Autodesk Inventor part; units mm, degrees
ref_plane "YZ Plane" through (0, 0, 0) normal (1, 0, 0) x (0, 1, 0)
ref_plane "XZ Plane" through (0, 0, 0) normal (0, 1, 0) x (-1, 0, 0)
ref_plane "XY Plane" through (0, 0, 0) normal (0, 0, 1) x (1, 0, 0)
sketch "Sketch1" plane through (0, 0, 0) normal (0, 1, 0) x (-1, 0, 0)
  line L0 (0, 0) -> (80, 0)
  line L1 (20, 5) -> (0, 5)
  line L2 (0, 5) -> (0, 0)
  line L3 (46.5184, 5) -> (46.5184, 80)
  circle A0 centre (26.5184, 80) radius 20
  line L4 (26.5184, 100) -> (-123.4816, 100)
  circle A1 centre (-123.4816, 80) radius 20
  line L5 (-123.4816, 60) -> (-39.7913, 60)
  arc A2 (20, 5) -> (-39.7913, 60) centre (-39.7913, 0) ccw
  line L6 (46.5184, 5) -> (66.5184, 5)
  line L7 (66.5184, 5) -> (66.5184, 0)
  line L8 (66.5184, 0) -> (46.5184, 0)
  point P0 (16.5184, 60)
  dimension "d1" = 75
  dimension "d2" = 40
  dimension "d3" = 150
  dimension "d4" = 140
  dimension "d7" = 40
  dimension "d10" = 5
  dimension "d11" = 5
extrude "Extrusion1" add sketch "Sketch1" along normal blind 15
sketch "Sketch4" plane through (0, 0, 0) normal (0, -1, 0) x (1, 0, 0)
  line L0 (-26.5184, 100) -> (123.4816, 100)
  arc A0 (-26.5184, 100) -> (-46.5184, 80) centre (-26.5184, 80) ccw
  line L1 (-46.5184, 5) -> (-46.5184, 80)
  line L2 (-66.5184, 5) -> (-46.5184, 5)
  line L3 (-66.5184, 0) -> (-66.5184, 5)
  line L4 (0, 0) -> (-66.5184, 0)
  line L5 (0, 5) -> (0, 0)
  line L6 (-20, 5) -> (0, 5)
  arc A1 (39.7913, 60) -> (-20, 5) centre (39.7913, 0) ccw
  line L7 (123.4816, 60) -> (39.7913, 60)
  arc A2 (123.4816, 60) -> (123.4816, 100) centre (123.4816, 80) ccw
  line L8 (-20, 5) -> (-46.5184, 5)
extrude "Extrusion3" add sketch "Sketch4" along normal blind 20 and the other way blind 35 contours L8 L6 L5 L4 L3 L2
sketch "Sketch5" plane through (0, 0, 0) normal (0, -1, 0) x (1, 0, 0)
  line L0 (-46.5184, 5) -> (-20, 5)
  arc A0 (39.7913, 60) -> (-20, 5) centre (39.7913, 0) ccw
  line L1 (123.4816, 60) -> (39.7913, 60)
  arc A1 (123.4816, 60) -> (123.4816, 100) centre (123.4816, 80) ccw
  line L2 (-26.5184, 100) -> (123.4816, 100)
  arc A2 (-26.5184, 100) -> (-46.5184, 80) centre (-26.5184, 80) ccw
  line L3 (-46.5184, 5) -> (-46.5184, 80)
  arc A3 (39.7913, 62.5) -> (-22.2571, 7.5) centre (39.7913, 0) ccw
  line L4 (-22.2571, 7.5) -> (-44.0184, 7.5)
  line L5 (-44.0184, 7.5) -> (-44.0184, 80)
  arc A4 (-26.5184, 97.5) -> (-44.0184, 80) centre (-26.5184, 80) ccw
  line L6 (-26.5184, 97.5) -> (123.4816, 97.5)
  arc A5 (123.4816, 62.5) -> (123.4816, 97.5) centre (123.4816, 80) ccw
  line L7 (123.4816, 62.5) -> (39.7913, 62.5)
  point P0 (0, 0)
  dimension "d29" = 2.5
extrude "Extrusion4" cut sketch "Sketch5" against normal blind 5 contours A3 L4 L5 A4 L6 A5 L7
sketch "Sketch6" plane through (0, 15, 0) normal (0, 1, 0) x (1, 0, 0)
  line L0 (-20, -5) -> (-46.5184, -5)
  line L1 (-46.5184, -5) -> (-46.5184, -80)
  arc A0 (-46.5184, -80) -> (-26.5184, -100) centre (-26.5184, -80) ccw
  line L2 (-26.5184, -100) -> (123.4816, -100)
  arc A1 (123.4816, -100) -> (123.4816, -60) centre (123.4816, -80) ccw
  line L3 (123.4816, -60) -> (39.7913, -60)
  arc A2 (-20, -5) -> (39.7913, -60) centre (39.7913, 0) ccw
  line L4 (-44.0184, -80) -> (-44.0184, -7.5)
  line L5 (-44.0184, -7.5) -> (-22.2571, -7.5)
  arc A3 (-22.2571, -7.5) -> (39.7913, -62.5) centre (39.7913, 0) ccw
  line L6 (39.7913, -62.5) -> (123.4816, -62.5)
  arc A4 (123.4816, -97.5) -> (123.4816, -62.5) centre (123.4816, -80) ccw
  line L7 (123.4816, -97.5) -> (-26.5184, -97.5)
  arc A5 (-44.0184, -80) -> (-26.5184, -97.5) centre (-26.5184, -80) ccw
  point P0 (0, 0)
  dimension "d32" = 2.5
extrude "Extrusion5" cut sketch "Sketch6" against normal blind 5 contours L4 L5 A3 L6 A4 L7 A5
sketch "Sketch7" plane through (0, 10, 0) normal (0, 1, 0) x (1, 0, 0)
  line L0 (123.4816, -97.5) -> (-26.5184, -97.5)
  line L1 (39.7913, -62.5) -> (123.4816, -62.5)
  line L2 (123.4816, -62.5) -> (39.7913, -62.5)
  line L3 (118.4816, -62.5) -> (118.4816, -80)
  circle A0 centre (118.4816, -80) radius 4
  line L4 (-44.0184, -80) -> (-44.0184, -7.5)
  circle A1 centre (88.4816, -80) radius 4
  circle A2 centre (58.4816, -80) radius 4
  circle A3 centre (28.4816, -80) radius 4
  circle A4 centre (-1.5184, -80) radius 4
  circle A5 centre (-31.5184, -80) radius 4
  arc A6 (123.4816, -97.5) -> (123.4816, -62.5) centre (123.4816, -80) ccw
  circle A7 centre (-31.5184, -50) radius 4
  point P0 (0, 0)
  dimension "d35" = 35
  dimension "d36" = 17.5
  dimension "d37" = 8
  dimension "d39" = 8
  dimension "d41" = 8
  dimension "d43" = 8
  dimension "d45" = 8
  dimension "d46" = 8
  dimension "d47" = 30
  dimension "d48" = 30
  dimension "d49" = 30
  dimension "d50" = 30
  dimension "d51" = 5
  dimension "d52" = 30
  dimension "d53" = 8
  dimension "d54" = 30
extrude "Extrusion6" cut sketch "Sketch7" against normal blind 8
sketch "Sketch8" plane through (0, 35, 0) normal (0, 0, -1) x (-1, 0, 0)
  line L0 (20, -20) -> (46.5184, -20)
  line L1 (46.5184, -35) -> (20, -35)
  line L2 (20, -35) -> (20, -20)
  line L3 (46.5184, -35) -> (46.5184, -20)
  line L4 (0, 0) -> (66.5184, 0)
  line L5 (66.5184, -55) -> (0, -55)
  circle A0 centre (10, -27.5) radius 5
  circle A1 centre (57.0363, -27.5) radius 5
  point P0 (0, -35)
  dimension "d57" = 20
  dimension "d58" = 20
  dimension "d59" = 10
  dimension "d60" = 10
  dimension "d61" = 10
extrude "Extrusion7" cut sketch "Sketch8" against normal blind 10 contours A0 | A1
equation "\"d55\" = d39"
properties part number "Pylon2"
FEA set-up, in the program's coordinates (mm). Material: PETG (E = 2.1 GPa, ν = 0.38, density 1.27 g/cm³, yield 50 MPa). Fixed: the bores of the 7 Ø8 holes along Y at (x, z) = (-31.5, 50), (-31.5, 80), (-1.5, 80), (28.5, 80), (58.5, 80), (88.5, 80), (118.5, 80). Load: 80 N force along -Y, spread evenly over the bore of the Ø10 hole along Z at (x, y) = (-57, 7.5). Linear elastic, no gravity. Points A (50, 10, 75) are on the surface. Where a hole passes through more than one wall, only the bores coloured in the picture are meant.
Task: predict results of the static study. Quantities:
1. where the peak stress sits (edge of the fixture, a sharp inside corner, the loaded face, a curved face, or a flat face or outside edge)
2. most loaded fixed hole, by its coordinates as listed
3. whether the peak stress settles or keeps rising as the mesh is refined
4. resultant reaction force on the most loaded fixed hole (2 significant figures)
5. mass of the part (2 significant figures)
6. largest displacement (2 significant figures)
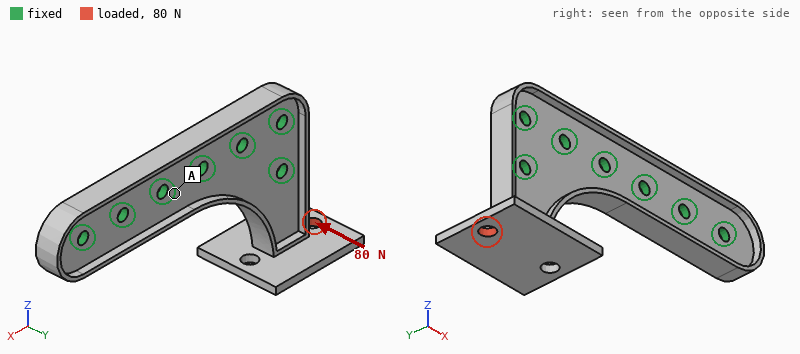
edge of the fixture
(-31.5, 50)
keeps rising
160 N
97 g
2.7 mm
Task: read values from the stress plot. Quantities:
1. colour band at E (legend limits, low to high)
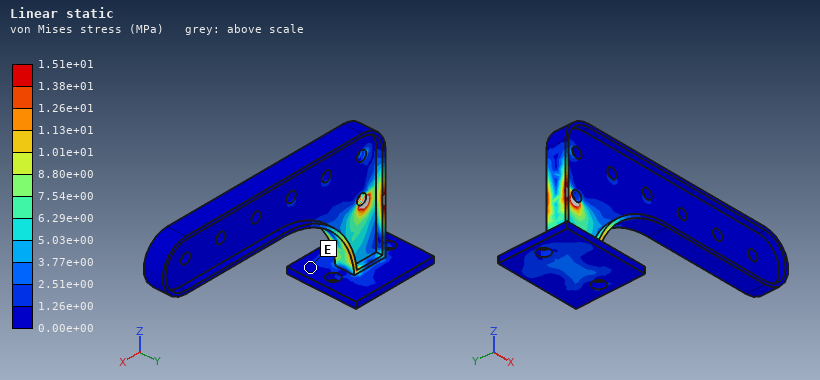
0.00e+00 to 1.26e+00 MPa
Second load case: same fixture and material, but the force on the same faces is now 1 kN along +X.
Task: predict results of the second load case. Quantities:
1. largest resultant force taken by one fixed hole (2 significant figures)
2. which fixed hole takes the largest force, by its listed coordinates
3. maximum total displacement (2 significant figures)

1.2 kN
(-31.5, 50)
1.6 mm
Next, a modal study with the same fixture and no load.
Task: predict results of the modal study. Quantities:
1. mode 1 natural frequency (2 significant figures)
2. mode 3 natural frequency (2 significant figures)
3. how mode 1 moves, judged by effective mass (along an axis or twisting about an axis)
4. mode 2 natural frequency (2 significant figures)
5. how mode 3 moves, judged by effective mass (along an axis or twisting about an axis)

230 Hz
840 Hz
along Y
300 Hz
along X
